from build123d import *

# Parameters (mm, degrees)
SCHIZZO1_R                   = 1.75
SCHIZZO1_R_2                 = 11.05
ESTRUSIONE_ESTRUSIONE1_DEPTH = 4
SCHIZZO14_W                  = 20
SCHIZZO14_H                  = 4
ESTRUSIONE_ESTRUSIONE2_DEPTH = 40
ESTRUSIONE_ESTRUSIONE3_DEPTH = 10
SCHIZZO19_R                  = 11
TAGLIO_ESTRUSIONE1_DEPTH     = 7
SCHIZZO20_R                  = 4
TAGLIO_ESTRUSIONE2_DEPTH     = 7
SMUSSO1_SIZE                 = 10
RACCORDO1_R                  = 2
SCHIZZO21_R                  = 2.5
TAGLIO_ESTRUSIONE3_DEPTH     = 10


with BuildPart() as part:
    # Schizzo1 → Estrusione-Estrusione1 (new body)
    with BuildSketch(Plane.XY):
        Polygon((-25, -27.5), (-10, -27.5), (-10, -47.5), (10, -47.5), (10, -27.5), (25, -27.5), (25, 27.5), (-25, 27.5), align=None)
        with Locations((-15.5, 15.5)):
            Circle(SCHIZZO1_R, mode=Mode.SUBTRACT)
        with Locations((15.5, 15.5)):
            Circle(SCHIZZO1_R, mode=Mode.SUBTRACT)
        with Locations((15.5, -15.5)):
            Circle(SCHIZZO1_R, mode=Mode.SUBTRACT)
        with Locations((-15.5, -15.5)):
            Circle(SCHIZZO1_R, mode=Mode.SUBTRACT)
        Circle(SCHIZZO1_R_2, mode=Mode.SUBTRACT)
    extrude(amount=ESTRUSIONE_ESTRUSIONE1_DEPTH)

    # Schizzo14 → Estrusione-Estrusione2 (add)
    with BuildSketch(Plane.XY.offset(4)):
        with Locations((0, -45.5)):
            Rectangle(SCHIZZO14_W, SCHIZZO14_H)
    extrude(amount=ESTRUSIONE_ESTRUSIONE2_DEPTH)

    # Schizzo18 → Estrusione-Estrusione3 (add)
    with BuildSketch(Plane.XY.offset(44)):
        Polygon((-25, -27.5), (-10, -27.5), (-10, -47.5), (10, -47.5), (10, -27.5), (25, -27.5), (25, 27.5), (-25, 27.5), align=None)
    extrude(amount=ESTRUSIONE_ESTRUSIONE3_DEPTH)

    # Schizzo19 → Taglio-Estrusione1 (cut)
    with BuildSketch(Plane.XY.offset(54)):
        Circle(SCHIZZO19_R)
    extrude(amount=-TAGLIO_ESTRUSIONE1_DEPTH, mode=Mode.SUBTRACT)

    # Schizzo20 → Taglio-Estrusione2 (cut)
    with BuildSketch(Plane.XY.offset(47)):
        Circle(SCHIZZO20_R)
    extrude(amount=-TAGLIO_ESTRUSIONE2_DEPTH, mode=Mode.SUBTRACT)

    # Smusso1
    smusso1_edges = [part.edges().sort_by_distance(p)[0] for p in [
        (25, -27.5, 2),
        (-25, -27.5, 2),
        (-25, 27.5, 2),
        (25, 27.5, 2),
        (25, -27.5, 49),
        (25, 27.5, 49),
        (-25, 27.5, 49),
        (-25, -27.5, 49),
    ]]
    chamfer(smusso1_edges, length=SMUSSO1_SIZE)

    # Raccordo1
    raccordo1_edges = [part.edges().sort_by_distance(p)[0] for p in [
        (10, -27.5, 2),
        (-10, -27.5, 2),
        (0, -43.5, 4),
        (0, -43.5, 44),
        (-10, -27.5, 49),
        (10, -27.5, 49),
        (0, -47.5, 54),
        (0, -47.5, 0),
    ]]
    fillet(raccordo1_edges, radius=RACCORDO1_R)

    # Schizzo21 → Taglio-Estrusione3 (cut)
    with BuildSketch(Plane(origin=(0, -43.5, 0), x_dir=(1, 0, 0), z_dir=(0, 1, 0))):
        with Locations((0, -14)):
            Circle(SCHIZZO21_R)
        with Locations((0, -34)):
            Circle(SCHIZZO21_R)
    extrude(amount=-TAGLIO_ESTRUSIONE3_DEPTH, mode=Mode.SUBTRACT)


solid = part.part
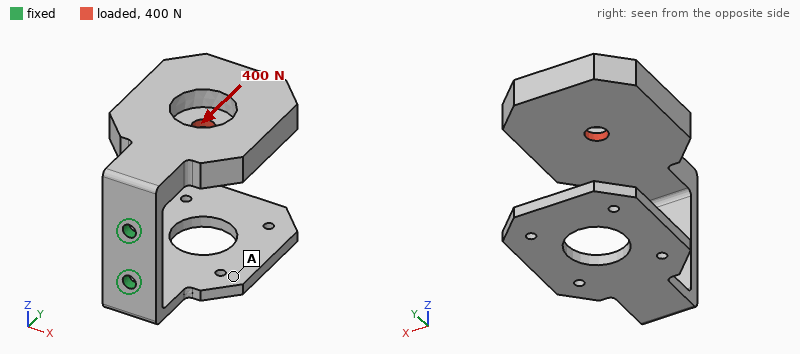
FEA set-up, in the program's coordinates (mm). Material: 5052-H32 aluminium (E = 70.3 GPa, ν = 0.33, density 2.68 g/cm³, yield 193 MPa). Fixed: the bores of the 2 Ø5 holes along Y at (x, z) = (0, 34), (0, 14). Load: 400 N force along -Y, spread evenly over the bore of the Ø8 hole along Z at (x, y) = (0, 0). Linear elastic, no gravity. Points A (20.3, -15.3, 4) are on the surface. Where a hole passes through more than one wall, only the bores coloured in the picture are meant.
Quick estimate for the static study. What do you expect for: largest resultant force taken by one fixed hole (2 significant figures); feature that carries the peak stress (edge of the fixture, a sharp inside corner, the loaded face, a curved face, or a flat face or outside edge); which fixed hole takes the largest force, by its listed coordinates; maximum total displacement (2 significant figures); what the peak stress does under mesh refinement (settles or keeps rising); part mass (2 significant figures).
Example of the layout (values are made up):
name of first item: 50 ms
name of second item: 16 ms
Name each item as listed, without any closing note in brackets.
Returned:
largest resultant force taken by one fixed hole: 440 N
feature that carries the peak stress: edge of the fixture
which fixed hole takes the largest force, by its listed coordinates: (0, 34)
maximum total displacement: 0.20 mm
what the peak stress does under mesh refinement: keeps rising
part mass: 110 g
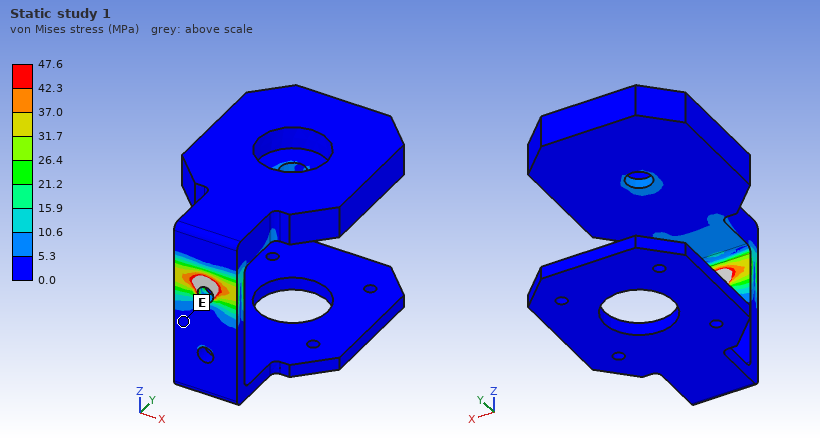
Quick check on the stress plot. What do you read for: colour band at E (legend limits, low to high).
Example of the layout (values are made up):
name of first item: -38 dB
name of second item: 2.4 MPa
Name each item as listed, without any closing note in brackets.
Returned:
colour band at E: 0.0 to 5.3 MPa
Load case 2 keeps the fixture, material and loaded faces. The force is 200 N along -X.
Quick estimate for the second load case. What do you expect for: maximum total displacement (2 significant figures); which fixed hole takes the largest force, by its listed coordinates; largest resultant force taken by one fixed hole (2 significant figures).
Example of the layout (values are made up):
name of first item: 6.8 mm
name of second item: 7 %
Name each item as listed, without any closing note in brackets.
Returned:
maximum total displacement: 0.48 mm
which fixed hole takes the largest force, by its listed coordinates: (0, 34)
largest resultant force taken by one fixed hole: 270 N
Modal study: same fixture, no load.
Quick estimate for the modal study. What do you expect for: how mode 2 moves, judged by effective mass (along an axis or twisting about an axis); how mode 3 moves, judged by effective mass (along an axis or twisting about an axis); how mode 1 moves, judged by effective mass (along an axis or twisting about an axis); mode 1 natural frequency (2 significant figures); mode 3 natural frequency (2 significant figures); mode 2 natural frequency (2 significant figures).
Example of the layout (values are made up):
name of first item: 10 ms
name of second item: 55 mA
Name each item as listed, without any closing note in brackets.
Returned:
how mode 2 moves, judged by effective mass: along Z
how mode 3 moves, judged by effective mass: along X
how mode 1 moves, judged by effective mass: along Z
mode 1 natural frequency: 340 Hz
mode 3 natural frequency: 480 Hz
mode 2 natural frequency: 390 Hz
